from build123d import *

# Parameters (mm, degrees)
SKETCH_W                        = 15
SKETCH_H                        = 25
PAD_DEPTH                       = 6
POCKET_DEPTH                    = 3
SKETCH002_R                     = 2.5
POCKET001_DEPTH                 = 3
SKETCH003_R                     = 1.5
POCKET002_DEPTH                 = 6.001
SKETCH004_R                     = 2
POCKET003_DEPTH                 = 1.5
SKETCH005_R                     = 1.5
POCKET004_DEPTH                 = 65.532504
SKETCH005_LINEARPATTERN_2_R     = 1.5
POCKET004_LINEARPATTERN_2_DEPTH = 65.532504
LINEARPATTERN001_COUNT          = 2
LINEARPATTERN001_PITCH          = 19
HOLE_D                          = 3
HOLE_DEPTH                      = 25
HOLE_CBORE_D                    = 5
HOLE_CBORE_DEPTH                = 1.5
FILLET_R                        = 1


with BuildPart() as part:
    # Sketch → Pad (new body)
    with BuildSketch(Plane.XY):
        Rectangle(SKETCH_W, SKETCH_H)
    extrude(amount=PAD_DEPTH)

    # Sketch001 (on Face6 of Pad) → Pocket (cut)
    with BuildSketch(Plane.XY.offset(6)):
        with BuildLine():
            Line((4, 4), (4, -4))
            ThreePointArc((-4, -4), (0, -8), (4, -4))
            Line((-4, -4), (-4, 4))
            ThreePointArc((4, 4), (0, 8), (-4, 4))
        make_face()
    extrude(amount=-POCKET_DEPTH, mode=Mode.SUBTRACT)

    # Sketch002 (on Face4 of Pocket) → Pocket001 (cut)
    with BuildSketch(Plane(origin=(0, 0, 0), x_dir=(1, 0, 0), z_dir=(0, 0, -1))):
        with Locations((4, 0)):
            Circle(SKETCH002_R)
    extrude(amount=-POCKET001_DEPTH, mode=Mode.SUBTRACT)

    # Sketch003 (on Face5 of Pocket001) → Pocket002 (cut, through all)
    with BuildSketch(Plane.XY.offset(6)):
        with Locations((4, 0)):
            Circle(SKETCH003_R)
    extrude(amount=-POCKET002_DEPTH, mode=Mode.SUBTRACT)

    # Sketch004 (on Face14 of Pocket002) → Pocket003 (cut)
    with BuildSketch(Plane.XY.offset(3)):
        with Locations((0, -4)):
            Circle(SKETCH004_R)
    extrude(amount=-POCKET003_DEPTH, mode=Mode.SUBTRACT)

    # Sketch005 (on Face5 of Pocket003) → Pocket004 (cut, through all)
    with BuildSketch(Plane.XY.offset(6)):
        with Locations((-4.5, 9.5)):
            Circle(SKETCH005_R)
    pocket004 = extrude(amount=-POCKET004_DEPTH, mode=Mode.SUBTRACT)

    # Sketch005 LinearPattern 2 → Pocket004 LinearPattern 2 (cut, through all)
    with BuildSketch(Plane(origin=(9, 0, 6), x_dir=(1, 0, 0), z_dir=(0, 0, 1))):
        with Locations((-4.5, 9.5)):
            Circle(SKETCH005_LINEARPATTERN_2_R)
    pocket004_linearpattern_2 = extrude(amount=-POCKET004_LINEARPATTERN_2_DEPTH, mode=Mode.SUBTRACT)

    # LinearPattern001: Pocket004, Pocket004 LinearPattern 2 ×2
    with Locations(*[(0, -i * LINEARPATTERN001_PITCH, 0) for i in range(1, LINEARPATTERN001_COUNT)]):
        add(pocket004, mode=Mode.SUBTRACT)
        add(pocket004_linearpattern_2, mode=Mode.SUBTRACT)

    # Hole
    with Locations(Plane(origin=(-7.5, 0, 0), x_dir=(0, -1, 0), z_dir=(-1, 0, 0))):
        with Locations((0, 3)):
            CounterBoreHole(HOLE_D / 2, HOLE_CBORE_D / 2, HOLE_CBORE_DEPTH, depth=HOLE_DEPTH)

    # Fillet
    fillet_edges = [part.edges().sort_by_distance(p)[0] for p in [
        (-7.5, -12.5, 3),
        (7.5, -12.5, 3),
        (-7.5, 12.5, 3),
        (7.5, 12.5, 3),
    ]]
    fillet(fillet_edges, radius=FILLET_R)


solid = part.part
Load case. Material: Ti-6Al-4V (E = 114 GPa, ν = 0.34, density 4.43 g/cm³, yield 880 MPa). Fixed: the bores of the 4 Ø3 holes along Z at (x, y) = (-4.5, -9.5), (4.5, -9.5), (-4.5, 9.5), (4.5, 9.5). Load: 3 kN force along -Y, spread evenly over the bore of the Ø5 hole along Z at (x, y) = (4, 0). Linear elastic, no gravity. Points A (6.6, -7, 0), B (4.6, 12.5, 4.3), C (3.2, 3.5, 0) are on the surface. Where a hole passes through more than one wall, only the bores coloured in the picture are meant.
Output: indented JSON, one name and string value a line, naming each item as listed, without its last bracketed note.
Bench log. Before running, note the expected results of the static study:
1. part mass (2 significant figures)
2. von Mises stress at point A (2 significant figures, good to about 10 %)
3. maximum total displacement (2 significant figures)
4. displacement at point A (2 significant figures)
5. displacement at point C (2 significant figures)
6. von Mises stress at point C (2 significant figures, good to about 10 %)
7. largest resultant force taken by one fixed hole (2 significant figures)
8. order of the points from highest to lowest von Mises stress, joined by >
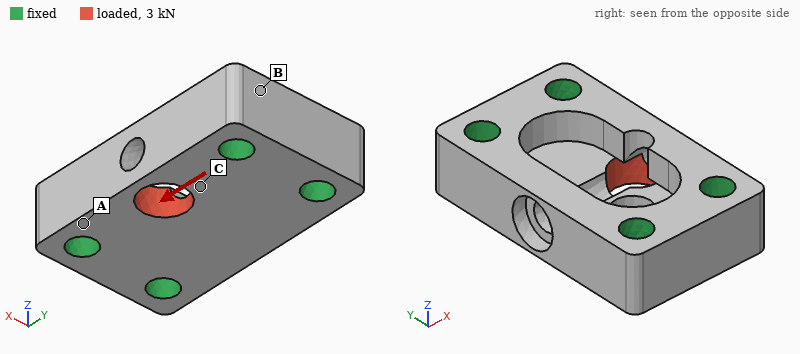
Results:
{
  "part mass": "6.9 g",
  "von Mises stress at point A": "50 MPa",
  "maximum total displacement": "5.0 µm",
  "displacement at point A": "1.4 µm",
  "displacement at point C": "3.1 µm",
  "von Mises stress at point C": "80 MPa",
  "largest resultant force taken by one fixed hole": "1.2 kN",
  "order of the points from highest to lowest von Mises stress, joined by >": "C > A > B"
}
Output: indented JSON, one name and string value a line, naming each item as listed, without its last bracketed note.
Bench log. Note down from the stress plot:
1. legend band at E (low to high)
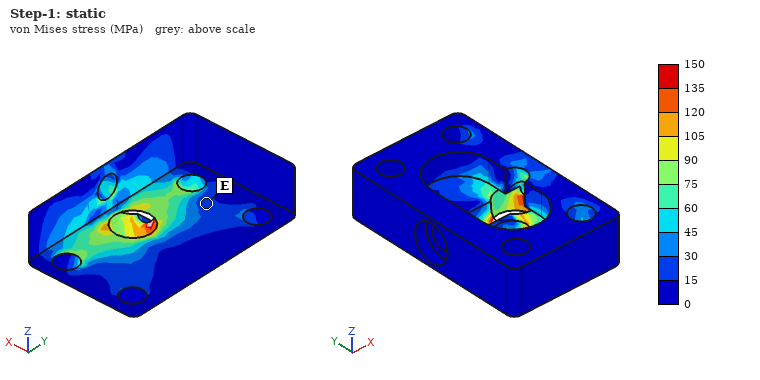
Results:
{
  "legend band at E": "15 to 30 MPa"
}
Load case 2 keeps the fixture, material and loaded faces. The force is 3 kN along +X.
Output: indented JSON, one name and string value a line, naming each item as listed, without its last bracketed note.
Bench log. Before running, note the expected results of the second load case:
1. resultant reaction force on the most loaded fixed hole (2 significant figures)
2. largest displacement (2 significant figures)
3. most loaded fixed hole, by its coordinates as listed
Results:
{
  "resultant reaction force on the most loaded fixed hole": "1.0 kN",
  "largest displacement": "20 µm",
  "most loaded fixed hole, by its coordinates as listed": "(-4.5, 9.5)"
}
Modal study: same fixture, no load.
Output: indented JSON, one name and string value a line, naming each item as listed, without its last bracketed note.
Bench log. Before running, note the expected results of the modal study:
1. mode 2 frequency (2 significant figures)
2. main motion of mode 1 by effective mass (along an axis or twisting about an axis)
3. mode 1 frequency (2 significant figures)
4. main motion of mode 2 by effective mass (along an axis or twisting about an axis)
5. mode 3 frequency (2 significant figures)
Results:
{
  "mode 2 frequency": "75 kHz",
  "main motion of mode 1 by effective mass": "along Z",
  "mode 1 frequency": "67 kHz",
  "main motion of mode 2 by effective mass": "along X",
  "mode 3 frequency": "82 kHz"
}
